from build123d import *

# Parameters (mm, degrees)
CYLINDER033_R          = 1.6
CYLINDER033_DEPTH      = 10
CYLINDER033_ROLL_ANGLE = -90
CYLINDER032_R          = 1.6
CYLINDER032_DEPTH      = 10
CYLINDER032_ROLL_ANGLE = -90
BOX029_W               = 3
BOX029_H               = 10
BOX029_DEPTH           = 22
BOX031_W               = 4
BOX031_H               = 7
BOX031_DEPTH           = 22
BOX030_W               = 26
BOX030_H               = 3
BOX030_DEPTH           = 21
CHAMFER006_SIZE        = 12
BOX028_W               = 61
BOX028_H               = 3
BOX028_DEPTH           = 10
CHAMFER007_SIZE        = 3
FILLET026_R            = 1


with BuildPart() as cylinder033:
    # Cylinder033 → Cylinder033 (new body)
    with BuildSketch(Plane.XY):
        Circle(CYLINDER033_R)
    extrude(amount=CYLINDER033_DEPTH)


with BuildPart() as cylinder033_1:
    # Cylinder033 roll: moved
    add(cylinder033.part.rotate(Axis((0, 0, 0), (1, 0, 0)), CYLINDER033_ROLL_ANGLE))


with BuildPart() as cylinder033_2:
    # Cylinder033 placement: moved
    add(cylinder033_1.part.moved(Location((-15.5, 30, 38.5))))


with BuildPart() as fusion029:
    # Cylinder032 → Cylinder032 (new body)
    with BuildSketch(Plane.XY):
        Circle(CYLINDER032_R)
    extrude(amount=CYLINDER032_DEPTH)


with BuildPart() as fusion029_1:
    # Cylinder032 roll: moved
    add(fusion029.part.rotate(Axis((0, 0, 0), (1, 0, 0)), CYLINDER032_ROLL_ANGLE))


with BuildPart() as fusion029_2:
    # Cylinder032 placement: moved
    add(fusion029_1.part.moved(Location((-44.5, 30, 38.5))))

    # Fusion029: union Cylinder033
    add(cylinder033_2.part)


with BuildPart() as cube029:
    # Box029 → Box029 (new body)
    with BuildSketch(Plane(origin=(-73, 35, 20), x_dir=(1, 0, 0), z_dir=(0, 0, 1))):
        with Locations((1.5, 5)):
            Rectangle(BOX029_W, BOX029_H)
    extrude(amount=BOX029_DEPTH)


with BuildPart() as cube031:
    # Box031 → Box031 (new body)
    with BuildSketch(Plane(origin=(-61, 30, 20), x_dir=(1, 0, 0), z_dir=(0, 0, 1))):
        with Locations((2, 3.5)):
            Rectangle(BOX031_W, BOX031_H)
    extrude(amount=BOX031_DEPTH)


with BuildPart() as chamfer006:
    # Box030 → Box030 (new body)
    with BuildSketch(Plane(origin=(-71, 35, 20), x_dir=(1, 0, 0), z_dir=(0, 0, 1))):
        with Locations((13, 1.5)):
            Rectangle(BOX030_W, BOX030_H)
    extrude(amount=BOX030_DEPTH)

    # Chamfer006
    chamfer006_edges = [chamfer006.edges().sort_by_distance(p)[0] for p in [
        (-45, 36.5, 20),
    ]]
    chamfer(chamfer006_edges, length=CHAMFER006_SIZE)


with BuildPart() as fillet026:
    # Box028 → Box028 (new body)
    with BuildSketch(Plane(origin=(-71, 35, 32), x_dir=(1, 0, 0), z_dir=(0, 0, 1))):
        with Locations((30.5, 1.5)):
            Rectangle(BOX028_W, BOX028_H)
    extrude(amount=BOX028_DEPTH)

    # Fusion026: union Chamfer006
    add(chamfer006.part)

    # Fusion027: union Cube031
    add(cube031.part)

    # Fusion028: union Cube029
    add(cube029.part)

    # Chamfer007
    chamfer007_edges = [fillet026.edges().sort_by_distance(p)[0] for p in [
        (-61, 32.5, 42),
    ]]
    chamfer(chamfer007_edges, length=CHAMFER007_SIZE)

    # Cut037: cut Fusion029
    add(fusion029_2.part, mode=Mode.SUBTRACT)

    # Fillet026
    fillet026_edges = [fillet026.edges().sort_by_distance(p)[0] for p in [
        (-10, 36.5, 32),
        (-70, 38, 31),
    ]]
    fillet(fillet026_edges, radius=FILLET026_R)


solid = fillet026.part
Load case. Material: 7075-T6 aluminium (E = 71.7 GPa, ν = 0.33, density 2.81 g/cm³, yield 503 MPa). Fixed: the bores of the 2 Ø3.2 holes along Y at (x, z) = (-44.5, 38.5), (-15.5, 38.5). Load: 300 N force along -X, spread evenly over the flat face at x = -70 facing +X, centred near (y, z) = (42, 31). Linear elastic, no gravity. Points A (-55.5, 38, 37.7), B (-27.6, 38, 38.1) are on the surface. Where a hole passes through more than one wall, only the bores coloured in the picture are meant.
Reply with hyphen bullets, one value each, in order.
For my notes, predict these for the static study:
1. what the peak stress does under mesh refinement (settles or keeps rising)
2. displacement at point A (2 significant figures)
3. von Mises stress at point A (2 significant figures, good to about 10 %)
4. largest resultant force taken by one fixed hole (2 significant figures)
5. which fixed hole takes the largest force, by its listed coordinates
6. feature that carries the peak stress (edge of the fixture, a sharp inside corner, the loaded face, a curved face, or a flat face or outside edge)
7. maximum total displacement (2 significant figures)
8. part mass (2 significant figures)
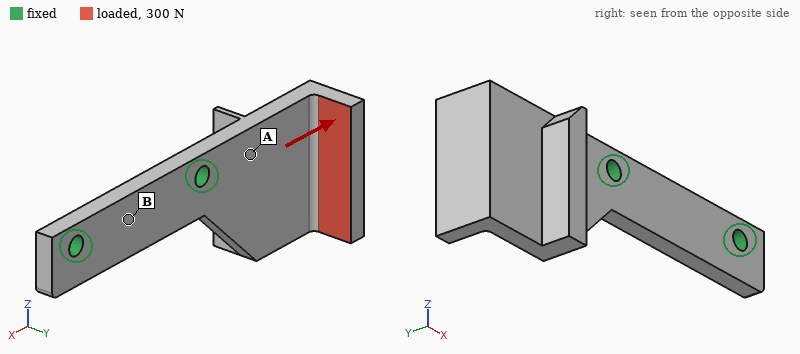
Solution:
- keeps rising
- 0.050 mm
- 66 MPa
- 230 N
- (-44.5, 38.5)
- edge of the fixture
- 0.32 mm
- 9.9 g
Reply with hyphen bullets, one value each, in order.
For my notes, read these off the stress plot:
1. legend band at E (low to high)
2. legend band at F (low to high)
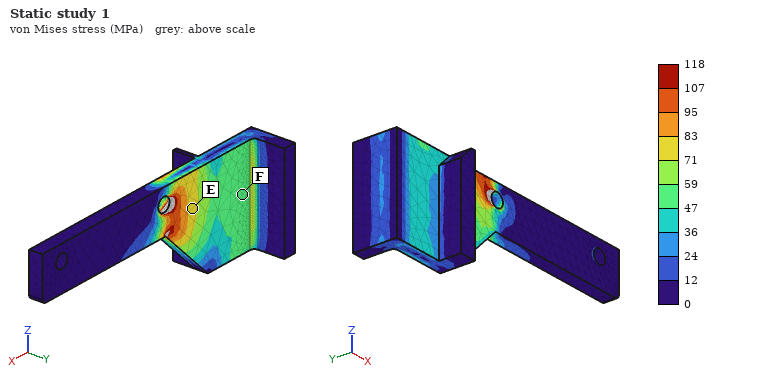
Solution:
- 71 to 83 MPa
- 47 to 59 MPa
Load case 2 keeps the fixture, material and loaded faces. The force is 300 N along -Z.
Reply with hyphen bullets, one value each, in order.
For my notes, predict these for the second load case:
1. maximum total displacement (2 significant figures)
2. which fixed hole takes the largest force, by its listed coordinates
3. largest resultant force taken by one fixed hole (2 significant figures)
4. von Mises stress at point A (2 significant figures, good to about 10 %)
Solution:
- 0.26 mm
- (-44.5, 38.5)
- 480 N
- 84 MPa
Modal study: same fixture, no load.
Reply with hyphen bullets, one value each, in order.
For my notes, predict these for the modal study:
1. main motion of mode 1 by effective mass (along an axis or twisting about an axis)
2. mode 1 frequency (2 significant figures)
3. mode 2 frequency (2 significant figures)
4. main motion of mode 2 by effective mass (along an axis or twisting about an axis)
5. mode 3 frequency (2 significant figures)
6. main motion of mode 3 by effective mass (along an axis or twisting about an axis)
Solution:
- along Y
- 1600 Hz
- 3900 Hz
- along Z
- 4600 Hz
- along Z
